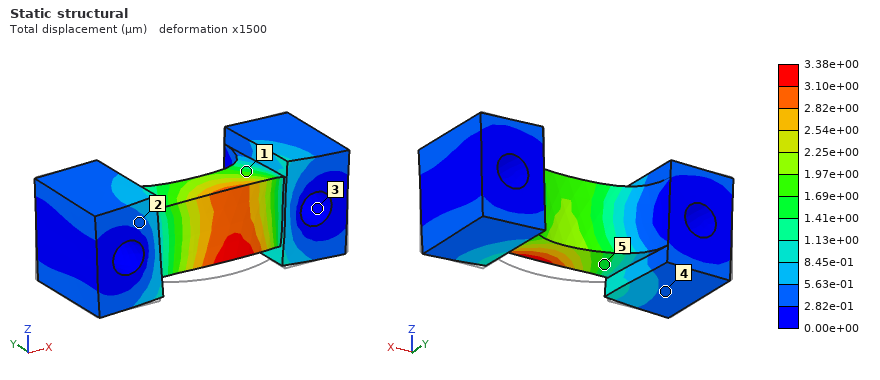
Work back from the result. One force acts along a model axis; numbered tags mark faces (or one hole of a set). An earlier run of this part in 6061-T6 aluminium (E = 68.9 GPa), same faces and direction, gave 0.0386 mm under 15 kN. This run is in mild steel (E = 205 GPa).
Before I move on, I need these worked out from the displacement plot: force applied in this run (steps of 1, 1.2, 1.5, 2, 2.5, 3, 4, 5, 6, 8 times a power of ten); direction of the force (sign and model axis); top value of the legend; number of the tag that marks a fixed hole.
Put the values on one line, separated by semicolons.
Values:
4 kN; +Z; 3.38e+00 µm; 3
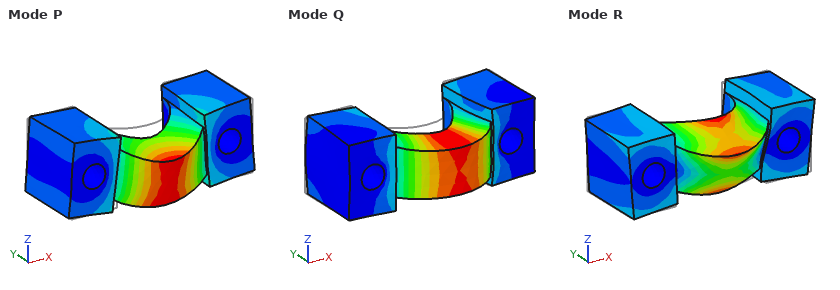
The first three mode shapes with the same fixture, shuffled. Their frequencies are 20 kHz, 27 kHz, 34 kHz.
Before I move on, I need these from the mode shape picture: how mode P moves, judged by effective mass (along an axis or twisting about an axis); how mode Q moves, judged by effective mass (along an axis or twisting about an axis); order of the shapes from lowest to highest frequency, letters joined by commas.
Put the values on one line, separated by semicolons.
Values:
along Z; along Y; P, Q, R
